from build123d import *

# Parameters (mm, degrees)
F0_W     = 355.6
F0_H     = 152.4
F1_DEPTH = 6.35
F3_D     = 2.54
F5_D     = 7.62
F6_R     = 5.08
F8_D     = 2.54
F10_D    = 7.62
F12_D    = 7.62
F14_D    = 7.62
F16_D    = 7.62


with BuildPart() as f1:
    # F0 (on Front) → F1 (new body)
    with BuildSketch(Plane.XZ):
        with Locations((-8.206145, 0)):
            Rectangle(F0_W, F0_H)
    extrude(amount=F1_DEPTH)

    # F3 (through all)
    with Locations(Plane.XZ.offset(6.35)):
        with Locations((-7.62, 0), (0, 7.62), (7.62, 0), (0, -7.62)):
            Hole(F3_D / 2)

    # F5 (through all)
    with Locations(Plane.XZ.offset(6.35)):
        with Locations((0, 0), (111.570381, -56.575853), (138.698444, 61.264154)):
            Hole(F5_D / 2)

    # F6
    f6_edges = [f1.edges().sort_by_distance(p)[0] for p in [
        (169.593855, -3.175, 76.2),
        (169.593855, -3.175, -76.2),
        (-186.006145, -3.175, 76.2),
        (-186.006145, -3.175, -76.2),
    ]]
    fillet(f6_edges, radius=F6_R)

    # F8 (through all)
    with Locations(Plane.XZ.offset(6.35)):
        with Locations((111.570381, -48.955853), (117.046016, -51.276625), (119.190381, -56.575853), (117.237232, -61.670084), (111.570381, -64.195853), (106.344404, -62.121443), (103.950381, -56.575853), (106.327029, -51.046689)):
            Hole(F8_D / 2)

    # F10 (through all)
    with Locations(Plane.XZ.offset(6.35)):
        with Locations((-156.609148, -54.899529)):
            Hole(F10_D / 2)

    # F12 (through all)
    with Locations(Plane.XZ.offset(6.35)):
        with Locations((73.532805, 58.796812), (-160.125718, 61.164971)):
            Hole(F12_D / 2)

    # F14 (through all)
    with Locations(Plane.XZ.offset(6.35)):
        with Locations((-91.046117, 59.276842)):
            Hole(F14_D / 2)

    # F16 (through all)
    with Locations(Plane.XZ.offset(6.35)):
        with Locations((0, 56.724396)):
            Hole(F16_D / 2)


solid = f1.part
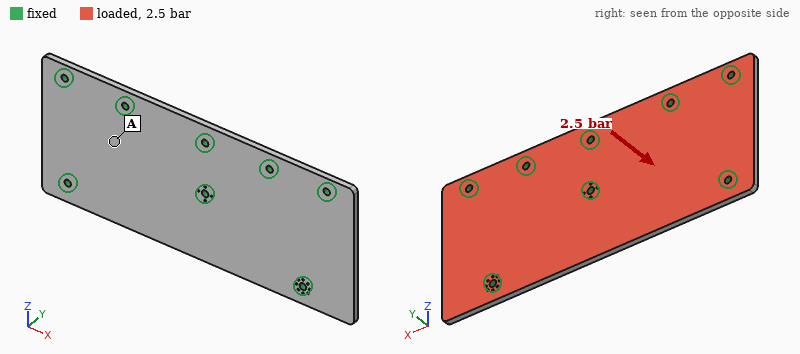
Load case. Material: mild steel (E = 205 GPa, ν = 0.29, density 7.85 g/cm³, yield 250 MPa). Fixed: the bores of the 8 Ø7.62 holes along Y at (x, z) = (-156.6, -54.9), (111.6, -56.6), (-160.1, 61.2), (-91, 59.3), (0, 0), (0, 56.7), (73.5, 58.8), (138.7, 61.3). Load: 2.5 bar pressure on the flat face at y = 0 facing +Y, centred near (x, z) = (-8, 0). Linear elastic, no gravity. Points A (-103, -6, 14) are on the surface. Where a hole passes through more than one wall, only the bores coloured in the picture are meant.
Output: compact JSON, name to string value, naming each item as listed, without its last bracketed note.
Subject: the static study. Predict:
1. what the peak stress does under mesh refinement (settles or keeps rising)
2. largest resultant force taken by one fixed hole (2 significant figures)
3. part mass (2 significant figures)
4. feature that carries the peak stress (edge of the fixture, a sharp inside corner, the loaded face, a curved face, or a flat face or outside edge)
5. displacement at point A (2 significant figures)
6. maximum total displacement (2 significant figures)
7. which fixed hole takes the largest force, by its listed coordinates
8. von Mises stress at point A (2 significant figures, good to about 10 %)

{"what the peak stress does under mesh refinement": "keeps rising", "largest resultant force taken by one fixed hole": "3.5 kN", "part mass": "2.7 kg", "feature that carries the peak stress": "a sharp inside corner", "displacement at point A": "0.055 mm", "maximum total displacement": "0.25 mm", "which fixed hole takes the largest force, by its listed coordinates": "(0, 0)", "von Mises stress at point A": "19 MPa"}
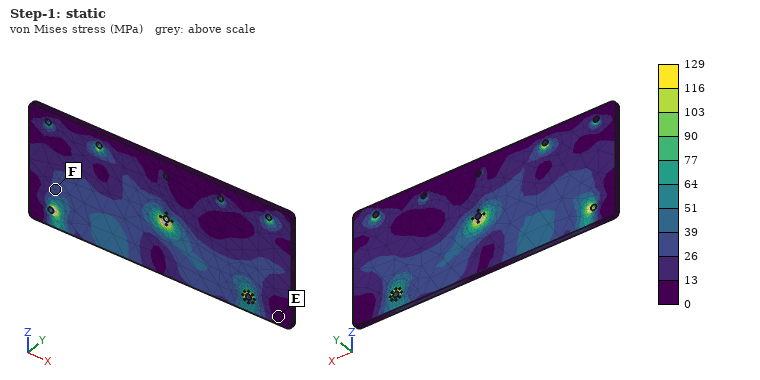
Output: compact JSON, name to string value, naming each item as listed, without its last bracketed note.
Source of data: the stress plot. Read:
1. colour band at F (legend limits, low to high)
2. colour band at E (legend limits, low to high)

{"colour band at F": "26 to 39 MPa", "colour band at E": "0 to 13 MPa"}
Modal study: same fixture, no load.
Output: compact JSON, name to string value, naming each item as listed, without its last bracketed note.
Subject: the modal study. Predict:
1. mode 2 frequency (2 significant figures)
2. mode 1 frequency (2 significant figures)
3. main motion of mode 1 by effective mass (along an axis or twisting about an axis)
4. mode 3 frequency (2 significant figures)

{"mode 2 frequency": "1400 Hz", "mode 1 frequency": "960 Hz", "main motion of mode 1 by effective mass": "along Y", "mode 3 frequency": "1600 Hz"}
